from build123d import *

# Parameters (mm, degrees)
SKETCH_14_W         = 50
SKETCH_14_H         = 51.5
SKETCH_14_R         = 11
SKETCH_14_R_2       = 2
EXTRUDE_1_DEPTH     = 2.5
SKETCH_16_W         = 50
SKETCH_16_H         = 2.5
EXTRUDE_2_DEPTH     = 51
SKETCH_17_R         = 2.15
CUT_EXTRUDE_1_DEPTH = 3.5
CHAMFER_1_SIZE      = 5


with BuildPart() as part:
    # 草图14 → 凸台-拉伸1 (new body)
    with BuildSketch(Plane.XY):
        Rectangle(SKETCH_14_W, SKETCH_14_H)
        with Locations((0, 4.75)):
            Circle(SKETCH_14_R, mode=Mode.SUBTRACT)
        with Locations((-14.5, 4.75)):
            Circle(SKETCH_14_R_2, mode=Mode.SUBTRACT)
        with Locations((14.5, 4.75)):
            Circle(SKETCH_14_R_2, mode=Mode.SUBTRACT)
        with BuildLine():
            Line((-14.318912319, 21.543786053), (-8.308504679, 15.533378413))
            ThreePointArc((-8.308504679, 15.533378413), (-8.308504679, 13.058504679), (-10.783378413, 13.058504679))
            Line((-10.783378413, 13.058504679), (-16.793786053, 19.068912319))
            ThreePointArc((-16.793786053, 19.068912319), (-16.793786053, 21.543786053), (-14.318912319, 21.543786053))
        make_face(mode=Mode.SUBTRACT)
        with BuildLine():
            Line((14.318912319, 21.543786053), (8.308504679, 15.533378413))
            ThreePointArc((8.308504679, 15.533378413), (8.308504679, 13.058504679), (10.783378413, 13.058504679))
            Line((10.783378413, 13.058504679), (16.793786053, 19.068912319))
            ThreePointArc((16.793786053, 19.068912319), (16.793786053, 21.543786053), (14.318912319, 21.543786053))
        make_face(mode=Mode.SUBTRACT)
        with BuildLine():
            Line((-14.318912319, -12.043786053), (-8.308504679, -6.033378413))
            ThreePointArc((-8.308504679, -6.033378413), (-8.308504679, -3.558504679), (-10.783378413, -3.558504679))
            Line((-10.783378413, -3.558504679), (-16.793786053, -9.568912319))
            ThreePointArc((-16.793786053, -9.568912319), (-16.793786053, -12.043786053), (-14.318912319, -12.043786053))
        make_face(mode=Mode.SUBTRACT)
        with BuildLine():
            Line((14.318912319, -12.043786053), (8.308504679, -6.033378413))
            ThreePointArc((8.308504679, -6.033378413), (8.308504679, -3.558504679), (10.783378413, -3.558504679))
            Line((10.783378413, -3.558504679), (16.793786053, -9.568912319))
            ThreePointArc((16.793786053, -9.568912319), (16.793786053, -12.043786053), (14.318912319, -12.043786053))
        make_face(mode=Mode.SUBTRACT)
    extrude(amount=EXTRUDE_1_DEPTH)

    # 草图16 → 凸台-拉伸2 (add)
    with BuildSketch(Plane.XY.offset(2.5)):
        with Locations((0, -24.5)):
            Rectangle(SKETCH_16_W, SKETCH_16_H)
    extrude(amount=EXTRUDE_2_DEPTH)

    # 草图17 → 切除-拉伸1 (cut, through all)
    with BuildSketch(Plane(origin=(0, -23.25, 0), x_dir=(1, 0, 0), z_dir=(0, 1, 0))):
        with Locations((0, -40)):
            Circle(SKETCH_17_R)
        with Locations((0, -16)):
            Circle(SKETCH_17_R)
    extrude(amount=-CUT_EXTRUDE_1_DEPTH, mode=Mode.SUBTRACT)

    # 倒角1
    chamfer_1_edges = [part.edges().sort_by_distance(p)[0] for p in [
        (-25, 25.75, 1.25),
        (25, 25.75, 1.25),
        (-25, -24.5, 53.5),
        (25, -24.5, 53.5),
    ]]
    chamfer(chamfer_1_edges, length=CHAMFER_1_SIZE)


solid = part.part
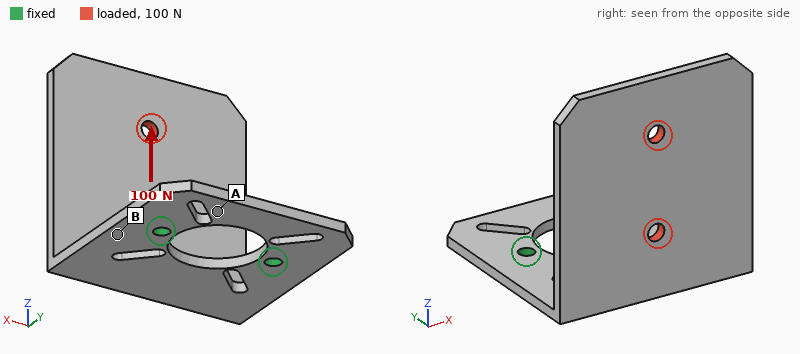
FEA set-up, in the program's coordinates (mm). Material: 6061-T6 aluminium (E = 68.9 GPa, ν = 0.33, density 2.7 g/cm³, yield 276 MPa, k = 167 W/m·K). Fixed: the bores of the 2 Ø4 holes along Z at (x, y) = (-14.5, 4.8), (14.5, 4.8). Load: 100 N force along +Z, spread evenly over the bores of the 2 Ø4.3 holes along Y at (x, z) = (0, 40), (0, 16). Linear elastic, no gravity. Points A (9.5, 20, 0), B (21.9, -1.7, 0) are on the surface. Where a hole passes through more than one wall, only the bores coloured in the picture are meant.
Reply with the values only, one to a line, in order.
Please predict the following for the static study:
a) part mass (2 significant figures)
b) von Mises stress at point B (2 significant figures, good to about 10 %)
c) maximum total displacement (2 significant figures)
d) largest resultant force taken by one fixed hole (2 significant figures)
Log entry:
30 g
69 MPa
0.93 mm
50 N
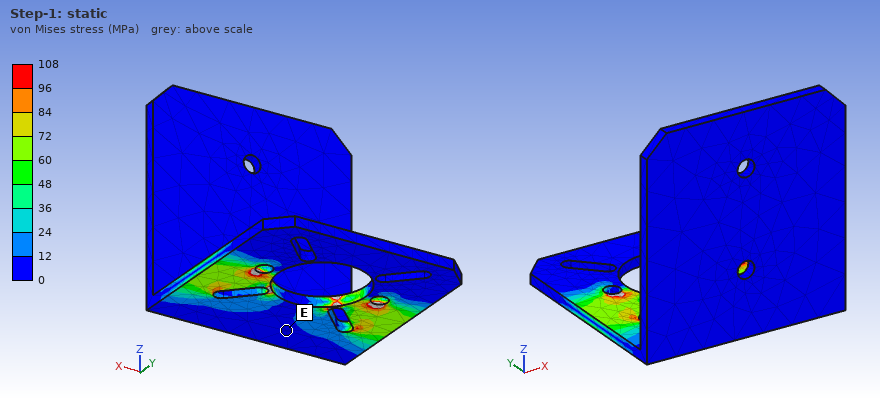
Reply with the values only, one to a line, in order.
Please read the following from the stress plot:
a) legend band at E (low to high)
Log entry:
0 to 12 MPa
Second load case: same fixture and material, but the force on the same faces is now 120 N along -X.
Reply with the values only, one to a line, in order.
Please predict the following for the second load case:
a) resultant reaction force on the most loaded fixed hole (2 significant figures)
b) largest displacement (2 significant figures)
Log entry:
130 N
0.43 mm
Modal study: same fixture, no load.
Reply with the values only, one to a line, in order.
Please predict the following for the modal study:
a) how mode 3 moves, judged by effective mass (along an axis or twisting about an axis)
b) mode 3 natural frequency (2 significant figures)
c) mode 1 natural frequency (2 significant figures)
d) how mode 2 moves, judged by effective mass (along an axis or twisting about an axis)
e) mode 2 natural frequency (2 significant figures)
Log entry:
along Z
1200 Hz
330 Hz
along X
730 Hz
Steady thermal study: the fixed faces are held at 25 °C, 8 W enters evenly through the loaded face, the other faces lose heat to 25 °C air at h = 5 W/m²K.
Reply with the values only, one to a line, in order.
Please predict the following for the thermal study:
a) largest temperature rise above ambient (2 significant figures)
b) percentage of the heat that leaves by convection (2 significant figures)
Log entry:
30 K
10 %
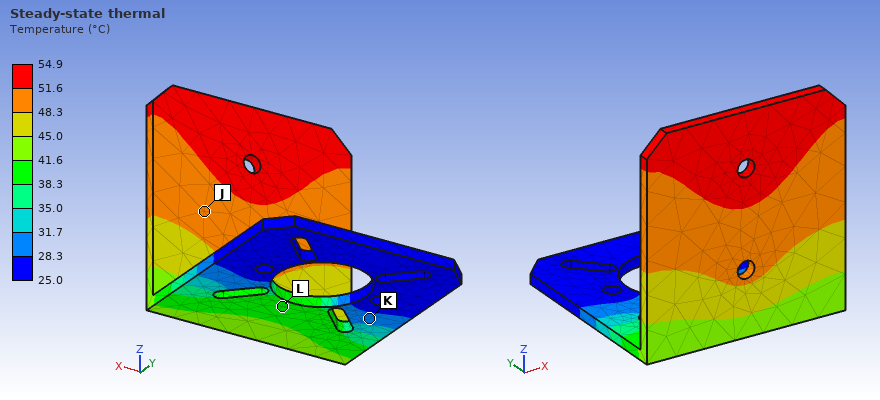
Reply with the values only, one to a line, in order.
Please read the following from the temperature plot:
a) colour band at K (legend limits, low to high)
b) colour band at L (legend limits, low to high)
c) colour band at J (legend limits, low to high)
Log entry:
28.3 to 31.7 °C
38.3 to 41.6 °C
48.3 to 51.6 °C
